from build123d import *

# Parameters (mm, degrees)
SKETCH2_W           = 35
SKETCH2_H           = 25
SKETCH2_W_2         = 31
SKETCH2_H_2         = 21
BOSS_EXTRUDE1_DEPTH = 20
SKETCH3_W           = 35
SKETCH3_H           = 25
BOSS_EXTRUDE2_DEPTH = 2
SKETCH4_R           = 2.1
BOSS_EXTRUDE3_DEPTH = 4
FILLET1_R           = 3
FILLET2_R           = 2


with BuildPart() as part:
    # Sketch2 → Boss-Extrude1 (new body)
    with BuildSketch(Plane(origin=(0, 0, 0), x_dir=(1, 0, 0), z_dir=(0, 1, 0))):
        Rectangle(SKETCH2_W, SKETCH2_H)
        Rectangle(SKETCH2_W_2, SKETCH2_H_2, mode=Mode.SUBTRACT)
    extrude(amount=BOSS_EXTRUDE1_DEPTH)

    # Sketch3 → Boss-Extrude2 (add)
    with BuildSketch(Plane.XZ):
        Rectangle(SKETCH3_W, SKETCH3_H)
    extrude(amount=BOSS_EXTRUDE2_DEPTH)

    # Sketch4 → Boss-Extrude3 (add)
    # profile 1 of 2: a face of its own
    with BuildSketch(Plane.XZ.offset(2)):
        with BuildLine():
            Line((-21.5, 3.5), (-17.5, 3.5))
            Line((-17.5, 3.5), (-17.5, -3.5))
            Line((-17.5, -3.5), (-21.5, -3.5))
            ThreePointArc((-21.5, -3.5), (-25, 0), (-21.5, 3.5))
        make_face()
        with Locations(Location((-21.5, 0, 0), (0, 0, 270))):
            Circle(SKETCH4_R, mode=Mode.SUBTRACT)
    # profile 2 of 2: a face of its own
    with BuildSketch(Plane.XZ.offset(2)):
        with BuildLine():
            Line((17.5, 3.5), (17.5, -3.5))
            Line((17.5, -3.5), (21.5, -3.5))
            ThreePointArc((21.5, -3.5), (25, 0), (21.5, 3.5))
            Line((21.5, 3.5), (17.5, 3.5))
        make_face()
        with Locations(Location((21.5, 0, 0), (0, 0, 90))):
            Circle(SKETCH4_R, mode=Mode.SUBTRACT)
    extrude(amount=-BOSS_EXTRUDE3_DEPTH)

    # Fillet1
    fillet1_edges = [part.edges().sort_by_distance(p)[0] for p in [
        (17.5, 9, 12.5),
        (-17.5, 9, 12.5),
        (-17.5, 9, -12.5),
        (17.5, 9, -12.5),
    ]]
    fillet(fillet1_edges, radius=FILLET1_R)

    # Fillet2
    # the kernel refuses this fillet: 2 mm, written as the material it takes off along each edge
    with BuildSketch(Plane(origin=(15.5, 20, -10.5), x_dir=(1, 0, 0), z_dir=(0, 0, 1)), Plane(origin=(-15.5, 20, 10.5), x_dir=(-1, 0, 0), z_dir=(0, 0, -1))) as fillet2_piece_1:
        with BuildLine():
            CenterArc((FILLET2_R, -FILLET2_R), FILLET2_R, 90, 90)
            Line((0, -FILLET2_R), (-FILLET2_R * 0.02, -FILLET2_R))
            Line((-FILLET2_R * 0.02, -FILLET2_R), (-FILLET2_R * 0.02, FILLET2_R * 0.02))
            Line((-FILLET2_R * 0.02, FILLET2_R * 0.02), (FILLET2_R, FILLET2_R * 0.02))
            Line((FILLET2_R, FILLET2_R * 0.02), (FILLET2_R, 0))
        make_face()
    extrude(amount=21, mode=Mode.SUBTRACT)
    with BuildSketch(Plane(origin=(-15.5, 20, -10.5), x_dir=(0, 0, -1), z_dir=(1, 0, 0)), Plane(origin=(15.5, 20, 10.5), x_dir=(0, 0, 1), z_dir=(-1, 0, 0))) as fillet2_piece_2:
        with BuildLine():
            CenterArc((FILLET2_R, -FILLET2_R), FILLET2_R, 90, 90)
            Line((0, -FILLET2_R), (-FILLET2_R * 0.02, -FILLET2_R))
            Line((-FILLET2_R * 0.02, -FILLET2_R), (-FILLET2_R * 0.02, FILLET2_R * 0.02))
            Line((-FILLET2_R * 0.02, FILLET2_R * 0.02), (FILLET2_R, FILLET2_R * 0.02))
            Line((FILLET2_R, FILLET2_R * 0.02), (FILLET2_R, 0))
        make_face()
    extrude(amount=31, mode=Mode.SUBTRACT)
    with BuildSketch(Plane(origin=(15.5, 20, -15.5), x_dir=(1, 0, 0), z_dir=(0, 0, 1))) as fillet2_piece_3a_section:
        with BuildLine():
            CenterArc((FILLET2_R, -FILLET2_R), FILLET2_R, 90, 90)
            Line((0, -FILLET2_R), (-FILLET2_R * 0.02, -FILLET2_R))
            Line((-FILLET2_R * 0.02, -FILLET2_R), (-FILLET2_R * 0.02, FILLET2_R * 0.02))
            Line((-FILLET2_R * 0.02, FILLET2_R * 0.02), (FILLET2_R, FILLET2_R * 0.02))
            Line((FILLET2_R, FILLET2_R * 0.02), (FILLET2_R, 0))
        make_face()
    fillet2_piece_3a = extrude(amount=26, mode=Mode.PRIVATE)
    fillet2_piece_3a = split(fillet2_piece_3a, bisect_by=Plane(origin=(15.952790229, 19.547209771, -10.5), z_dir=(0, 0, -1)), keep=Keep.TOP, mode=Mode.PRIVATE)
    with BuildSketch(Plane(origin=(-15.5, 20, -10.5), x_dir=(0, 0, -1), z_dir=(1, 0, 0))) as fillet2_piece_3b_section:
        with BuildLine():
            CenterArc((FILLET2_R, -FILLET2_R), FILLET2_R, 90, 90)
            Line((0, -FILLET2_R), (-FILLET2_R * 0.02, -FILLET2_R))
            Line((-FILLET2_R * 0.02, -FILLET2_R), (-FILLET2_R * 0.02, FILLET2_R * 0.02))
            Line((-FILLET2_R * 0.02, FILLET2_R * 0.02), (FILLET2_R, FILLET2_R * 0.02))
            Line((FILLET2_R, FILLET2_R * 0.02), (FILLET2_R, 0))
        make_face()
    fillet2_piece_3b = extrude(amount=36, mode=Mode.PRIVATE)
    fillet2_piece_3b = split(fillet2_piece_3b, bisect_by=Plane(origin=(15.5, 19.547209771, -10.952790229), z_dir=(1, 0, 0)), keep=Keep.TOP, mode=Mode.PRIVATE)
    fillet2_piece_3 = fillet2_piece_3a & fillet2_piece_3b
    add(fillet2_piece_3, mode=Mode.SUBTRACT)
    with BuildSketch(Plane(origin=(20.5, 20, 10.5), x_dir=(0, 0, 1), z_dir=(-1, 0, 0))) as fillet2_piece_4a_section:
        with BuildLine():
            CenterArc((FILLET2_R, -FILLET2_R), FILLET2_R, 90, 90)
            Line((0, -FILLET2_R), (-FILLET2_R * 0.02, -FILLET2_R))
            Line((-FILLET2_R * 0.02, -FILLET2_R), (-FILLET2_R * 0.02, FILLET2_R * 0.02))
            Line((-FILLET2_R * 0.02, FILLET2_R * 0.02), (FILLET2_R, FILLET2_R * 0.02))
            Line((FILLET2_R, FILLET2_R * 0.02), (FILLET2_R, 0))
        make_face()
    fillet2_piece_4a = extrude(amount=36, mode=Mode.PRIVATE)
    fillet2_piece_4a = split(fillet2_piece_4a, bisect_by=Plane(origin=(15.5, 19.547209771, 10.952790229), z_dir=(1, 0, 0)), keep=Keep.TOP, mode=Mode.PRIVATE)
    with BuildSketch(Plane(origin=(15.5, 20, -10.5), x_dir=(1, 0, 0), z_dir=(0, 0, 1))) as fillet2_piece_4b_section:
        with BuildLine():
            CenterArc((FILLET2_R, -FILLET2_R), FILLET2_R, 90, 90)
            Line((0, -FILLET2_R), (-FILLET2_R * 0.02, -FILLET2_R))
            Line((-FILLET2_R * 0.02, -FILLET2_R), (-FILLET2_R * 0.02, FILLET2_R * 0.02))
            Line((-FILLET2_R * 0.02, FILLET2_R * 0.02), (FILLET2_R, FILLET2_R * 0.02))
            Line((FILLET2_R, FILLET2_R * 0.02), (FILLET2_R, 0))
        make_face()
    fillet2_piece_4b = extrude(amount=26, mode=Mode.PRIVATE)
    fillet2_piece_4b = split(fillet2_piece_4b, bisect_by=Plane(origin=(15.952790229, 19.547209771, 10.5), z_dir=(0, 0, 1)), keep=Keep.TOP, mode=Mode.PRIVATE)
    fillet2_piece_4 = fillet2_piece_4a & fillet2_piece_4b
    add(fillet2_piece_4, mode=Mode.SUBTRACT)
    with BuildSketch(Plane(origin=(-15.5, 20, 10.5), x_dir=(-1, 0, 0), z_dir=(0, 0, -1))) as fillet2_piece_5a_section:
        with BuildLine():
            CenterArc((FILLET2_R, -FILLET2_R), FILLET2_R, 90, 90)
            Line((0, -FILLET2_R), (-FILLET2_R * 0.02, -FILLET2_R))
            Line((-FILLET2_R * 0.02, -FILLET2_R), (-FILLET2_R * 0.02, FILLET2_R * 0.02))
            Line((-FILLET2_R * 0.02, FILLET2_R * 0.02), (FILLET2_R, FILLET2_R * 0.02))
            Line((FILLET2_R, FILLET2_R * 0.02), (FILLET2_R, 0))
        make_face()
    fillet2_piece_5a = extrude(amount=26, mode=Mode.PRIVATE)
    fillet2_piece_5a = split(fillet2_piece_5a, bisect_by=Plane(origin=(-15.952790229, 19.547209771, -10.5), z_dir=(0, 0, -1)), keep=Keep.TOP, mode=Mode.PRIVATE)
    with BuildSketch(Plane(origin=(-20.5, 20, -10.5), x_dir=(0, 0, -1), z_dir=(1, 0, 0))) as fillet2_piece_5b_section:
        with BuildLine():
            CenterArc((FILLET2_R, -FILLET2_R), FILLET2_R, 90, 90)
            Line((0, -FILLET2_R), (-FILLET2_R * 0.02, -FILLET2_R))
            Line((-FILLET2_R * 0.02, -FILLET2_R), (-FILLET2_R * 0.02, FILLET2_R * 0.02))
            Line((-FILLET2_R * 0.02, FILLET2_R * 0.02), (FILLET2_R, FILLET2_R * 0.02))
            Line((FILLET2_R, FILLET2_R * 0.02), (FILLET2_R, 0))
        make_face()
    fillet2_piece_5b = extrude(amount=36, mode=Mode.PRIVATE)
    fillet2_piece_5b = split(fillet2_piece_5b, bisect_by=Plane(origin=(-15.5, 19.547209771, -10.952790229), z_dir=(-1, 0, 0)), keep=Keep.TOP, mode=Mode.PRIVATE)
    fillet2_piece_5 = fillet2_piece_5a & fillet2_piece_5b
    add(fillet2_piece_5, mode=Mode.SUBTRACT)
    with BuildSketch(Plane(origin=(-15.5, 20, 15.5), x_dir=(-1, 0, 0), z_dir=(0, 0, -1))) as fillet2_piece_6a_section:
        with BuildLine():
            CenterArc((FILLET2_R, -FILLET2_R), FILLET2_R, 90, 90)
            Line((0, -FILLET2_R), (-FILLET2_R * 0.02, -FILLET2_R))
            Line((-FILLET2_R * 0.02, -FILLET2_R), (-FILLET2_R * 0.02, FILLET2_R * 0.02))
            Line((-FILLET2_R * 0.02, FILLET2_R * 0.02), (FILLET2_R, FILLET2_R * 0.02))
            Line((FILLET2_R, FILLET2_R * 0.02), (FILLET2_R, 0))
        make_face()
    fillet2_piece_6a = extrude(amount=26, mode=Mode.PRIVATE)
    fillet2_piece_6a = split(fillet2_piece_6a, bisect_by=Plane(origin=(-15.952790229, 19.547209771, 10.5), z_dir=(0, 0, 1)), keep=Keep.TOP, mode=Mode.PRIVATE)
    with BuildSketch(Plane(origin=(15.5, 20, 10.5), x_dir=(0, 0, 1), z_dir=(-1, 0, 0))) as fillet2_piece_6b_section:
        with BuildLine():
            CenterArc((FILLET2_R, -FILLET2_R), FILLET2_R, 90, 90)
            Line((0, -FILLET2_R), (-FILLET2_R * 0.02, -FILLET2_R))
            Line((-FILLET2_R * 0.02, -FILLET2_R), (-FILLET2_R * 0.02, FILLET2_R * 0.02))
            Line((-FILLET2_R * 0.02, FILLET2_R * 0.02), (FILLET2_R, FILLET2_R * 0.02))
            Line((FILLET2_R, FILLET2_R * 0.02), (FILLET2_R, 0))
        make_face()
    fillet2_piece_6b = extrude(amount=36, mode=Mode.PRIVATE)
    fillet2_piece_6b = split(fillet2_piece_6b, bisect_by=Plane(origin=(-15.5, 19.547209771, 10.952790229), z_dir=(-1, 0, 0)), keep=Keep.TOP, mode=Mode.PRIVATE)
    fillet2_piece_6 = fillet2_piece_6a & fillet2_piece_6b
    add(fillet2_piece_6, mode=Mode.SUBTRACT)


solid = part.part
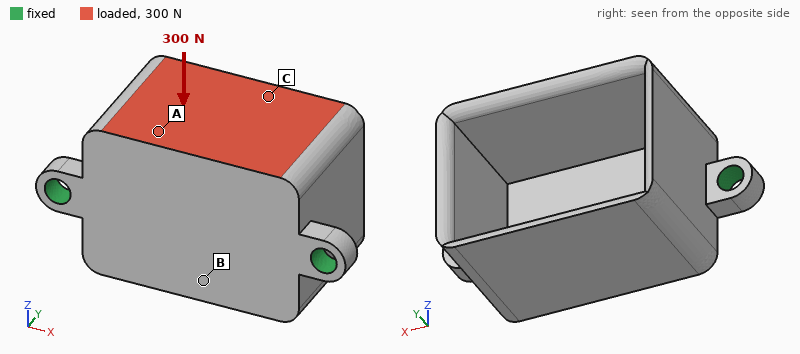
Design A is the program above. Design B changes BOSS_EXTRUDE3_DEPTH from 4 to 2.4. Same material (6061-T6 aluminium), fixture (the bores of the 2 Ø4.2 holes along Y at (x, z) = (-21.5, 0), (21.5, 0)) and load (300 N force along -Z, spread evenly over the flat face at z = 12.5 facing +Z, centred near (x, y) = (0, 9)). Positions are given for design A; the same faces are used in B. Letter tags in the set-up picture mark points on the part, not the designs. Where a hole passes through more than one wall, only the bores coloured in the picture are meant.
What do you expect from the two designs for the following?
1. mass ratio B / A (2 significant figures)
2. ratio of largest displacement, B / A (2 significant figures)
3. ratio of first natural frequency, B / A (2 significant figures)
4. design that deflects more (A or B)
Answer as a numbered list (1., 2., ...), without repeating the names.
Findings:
1. 0.98
2. 1.8
3. 0.62
4. B
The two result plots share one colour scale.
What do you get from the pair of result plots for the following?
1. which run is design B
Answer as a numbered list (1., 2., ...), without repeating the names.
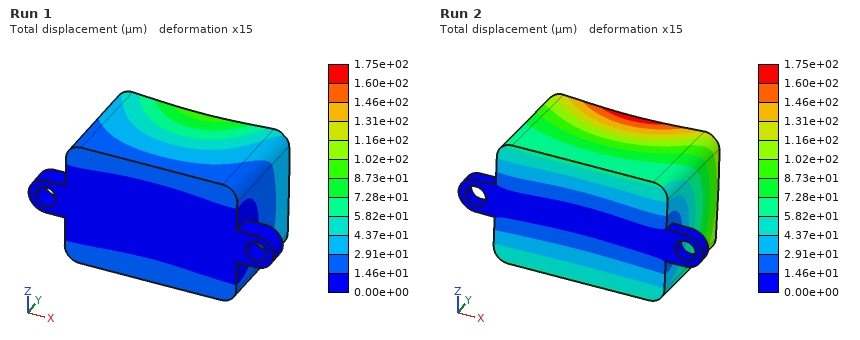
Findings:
1. Run 2
